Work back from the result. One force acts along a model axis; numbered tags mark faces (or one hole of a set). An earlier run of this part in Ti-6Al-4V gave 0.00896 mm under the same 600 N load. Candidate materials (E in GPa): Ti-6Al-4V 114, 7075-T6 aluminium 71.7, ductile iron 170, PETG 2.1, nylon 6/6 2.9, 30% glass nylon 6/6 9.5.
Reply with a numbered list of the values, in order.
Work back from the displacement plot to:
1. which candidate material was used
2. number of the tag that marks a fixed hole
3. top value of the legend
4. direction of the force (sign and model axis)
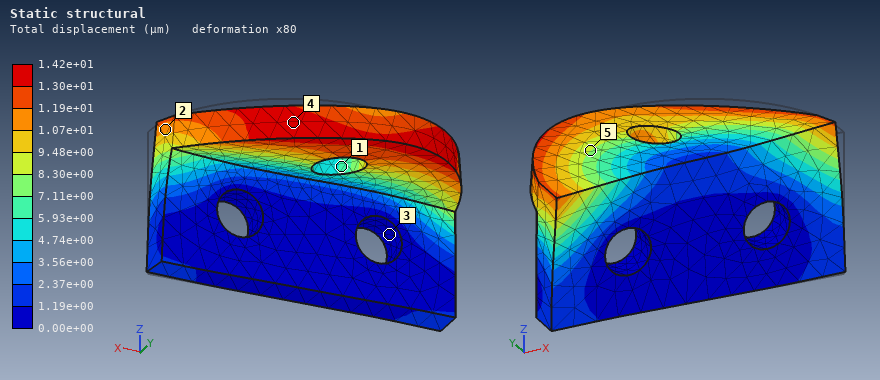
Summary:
1. 7075-T6 aluminium
2. 3
3. 1.42e+01 µm
4. -X
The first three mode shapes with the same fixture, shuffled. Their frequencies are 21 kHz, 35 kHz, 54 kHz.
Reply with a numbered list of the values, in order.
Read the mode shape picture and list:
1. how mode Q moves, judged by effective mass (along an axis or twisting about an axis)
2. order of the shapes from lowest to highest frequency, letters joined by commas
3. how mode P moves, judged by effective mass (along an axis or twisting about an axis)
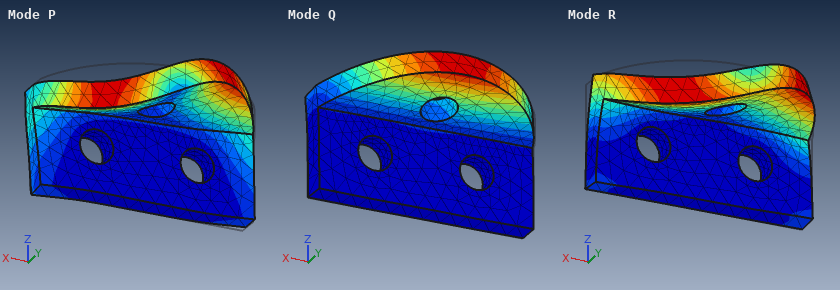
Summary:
1. along Z
2. Q, R, P
3. along X
